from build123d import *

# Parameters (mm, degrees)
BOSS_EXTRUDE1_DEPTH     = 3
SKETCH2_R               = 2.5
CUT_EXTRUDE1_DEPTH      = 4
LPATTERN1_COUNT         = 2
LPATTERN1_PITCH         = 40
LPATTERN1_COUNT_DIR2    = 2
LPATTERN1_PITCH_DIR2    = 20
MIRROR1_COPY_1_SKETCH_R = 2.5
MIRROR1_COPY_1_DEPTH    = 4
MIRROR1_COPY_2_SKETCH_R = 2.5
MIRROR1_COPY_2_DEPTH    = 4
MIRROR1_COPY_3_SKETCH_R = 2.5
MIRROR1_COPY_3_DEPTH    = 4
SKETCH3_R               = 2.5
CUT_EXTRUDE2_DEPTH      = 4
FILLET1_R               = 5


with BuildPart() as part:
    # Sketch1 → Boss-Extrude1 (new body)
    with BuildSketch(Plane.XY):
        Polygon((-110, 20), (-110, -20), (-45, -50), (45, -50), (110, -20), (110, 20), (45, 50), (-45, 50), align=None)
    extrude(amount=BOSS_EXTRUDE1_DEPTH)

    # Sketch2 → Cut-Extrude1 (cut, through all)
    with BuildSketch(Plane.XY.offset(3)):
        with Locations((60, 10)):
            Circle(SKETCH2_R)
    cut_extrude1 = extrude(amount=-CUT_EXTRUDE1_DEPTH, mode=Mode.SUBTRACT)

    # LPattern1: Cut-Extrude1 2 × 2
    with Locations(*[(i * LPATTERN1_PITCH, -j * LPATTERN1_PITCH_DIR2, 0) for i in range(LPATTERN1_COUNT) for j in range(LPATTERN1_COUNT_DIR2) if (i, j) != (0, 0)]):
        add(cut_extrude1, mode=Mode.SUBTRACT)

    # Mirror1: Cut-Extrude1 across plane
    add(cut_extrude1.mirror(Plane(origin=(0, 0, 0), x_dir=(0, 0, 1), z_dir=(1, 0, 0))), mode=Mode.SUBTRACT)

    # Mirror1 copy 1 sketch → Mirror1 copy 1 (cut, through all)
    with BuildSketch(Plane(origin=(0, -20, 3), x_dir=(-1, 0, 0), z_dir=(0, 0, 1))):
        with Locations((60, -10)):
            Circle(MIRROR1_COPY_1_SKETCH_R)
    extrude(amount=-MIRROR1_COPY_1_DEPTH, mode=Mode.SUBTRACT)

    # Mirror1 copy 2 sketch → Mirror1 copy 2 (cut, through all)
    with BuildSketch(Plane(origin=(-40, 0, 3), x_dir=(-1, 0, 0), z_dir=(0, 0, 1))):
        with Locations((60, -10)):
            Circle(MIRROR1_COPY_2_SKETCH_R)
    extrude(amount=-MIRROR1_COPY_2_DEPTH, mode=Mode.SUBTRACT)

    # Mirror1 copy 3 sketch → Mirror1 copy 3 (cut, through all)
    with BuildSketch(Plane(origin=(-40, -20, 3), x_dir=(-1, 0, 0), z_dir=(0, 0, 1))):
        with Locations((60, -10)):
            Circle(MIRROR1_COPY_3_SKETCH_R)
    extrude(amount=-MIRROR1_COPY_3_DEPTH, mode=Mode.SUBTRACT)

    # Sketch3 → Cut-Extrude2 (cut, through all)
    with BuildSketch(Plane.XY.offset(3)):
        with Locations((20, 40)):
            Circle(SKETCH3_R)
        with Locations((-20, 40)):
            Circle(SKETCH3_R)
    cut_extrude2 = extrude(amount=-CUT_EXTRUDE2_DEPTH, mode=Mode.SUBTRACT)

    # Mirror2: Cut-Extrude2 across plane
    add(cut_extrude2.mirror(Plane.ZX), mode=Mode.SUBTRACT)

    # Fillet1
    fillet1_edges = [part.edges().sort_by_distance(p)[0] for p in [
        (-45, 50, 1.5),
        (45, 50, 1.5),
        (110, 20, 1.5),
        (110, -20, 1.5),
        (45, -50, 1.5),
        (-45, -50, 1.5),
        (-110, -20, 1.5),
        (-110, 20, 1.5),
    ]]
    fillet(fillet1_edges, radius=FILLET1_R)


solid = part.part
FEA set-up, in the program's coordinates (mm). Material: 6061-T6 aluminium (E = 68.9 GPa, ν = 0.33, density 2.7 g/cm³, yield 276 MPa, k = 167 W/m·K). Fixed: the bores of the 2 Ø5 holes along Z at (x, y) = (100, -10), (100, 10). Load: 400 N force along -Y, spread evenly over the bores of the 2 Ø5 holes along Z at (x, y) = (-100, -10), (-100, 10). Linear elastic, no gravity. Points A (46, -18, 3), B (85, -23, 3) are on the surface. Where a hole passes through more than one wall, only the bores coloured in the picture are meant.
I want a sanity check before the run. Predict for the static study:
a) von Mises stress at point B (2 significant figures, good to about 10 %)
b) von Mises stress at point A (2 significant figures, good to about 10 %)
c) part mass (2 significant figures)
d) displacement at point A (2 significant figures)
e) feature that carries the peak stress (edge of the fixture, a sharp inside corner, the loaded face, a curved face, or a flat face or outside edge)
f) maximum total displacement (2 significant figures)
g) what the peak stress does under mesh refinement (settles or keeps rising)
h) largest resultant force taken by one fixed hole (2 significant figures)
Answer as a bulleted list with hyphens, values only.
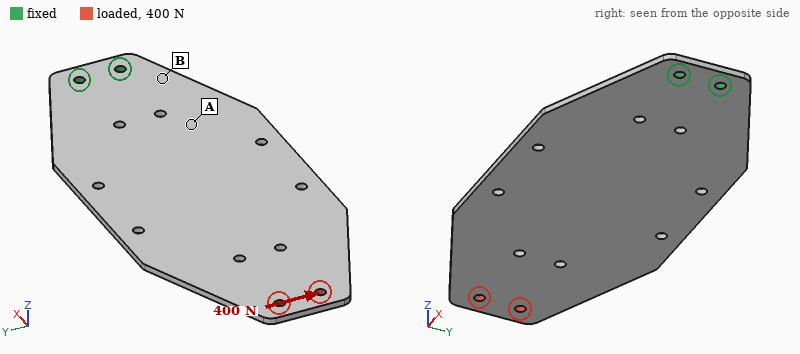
- 27 MPa
- 10 MPa
- 140 g
- 0.095 mm
- edge of the fixture
- 0.40 mm
- keeps rising
- 3.4 kN
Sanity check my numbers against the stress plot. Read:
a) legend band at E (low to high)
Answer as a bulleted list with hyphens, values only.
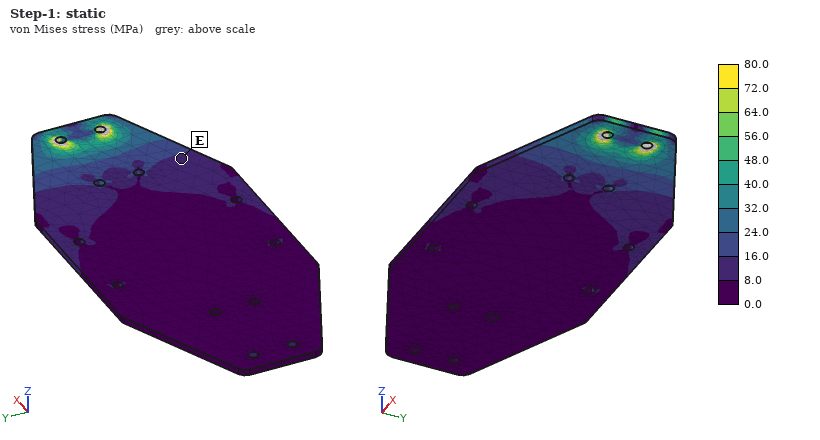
- 8.0 to 16.0 MPa
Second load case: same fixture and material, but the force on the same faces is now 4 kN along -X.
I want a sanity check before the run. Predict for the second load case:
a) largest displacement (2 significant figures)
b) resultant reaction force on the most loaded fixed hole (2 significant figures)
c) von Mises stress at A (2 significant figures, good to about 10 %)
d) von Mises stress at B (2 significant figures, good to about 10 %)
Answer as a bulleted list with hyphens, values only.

- 63 µm
- 2.0 kN
- 17 MPa
- 20 MPa
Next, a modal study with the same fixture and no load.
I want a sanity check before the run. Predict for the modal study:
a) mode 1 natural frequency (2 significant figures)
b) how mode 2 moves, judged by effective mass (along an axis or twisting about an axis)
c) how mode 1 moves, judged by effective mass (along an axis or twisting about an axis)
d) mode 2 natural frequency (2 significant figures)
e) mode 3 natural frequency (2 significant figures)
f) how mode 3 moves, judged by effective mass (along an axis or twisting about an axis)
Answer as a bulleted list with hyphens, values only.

- 57 Hz
- twisting about X
- along Z
- 260 Hz
- 350 Hz
- along Z
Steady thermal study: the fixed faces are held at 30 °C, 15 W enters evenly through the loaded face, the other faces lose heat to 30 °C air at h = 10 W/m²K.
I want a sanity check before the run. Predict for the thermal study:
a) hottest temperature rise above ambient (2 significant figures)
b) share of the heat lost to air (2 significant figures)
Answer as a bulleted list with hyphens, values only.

- 54 K
- 54 %
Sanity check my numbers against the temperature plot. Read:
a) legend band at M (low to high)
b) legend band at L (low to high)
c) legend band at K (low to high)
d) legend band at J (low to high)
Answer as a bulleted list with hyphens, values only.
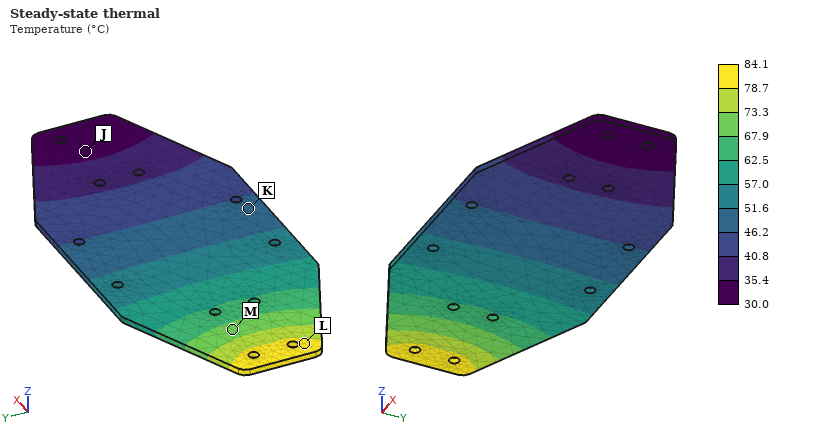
- 67.9 to 73.3 °C
- 78.7 to 84.1 °C
- 46.2 to 51.6 °C
- 30.0 to 35.4 °C
